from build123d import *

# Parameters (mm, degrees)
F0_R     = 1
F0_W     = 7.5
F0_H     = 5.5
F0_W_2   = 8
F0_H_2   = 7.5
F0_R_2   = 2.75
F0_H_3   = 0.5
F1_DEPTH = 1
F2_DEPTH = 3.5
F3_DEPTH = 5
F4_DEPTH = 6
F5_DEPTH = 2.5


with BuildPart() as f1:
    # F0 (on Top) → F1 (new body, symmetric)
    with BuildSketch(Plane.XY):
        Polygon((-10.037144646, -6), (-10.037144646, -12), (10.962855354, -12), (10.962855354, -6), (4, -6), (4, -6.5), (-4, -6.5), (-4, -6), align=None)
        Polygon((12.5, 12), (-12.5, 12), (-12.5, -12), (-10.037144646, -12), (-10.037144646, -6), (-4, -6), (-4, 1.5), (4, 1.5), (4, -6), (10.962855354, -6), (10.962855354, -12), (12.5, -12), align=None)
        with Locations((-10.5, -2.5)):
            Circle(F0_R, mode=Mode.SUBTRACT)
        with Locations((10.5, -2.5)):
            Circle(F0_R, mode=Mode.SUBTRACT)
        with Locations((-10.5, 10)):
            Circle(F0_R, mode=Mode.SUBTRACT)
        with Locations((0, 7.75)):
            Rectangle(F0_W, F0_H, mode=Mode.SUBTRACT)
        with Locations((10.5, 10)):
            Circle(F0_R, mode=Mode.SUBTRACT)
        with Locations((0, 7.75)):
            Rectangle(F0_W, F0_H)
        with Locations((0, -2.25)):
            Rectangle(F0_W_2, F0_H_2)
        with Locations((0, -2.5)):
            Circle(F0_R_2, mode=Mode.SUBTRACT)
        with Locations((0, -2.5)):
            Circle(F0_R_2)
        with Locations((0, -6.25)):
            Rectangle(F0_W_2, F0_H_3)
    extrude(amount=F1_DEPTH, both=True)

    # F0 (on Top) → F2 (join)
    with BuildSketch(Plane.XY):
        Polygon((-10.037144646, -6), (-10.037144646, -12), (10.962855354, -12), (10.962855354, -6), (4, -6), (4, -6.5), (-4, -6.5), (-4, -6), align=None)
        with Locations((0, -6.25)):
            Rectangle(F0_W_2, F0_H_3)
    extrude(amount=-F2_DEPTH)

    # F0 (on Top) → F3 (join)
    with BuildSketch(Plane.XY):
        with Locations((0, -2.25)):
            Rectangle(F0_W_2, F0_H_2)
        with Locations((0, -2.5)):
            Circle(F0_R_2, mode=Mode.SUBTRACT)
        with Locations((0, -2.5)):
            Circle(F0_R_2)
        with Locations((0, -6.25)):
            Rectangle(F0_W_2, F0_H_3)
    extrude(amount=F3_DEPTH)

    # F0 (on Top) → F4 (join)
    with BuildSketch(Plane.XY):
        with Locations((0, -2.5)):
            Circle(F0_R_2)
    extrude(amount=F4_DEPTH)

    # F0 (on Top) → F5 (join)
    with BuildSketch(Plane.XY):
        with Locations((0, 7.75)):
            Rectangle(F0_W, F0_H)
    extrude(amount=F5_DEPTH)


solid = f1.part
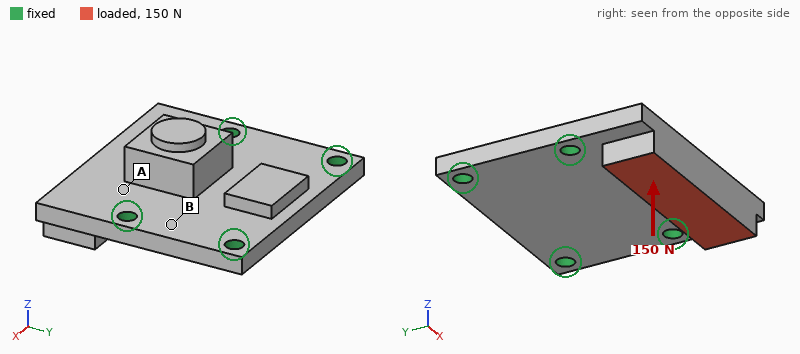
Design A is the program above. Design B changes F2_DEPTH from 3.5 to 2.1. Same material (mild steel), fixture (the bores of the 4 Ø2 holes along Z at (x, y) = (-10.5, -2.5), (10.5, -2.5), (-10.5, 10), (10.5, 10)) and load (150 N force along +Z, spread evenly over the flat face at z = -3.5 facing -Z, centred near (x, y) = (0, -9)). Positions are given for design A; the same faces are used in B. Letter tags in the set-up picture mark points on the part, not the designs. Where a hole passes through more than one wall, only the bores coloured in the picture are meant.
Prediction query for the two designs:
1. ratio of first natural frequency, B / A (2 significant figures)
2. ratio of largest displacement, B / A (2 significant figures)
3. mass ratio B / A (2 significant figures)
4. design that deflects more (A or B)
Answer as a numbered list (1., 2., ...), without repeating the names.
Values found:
1. 1.1
2. 1.1
3. 0.90
4. B
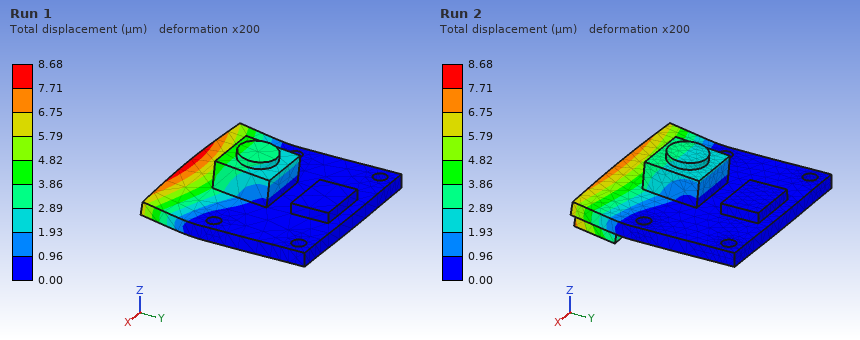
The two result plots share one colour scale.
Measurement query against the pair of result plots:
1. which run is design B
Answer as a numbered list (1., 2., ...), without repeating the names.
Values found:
1. Run 1
